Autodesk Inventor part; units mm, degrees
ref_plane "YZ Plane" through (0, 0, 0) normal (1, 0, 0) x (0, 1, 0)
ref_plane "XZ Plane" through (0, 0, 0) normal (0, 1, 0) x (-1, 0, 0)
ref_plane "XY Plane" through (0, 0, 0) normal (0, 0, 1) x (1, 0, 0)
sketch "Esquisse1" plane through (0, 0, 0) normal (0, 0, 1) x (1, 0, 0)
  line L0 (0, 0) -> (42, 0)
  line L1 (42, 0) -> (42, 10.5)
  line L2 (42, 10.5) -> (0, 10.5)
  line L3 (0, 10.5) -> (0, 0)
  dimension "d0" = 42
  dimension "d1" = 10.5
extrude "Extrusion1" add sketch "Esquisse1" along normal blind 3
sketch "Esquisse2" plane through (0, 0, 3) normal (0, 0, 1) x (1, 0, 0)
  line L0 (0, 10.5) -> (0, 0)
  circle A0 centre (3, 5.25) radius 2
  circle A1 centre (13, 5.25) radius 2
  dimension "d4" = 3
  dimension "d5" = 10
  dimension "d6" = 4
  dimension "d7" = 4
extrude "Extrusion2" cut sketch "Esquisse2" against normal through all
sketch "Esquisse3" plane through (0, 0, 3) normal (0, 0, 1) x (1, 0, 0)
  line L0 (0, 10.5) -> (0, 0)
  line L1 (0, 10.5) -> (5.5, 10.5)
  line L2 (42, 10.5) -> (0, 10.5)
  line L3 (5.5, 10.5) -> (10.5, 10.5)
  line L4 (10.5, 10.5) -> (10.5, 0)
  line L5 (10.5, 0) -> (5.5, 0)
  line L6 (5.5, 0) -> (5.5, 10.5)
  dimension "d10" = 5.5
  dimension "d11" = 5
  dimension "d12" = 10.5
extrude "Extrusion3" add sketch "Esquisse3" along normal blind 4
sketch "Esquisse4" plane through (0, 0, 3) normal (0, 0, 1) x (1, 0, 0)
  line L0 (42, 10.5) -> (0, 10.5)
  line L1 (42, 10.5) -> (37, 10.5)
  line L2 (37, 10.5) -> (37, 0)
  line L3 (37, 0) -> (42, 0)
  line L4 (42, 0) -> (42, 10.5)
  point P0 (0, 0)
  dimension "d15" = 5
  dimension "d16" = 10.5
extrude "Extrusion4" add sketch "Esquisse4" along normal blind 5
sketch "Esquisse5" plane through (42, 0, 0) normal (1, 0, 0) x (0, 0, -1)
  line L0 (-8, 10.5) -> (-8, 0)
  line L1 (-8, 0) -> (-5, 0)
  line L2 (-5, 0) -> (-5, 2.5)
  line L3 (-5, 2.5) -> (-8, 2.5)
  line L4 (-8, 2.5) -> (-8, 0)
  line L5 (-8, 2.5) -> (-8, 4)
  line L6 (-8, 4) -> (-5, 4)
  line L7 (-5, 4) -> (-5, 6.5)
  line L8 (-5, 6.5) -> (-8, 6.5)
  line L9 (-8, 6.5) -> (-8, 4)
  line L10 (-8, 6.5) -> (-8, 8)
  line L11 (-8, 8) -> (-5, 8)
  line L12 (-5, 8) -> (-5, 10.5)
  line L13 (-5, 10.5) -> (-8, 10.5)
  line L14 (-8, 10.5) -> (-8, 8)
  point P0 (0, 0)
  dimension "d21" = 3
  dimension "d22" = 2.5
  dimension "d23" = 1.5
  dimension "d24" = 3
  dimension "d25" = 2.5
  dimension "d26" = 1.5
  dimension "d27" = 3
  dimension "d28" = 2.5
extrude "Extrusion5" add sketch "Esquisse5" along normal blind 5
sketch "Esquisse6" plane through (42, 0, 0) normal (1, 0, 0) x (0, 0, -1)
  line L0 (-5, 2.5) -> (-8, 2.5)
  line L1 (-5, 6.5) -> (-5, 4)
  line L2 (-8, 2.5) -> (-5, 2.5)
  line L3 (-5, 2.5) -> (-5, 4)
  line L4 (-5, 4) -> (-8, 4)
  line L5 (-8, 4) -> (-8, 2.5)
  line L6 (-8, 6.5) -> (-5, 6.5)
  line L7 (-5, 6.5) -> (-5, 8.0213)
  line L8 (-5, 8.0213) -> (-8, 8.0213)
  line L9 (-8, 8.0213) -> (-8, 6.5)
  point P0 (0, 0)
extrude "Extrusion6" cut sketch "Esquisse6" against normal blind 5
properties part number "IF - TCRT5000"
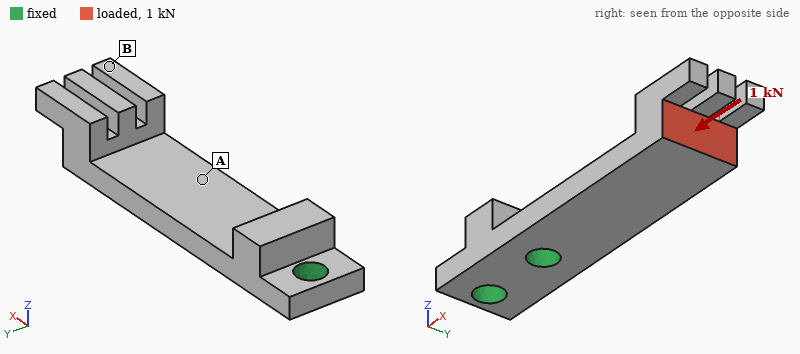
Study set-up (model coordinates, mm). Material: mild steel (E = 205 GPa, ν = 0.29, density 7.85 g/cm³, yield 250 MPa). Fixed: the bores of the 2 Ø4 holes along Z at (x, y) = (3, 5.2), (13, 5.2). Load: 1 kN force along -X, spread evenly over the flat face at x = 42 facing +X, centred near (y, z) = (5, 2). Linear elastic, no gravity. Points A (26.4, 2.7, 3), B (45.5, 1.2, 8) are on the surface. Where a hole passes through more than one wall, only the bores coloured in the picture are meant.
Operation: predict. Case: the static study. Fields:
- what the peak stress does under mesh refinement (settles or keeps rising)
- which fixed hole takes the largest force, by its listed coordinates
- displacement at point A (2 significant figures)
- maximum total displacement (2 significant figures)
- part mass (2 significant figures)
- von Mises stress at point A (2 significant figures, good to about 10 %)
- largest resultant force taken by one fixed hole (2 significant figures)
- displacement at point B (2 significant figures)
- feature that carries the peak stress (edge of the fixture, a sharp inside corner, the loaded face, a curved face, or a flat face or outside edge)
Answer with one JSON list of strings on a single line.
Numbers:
["keeps rising", "(13, 5.2)", "0.016 mm", "0.11 mm", "14 g", "95 MPa", "910 N", "0.10 mm", "edge of the fixture"]
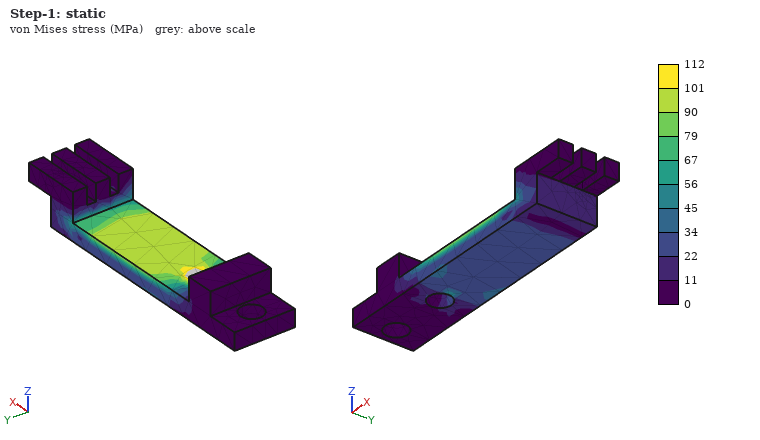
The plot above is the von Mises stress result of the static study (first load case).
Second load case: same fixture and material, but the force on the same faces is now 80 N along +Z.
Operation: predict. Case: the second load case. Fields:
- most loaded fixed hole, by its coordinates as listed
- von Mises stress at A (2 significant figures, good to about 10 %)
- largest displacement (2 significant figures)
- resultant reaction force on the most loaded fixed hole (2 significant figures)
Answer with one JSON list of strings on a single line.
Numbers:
["(13, 5.2)", "79 MPa", "0.15 mm", "98 N"]
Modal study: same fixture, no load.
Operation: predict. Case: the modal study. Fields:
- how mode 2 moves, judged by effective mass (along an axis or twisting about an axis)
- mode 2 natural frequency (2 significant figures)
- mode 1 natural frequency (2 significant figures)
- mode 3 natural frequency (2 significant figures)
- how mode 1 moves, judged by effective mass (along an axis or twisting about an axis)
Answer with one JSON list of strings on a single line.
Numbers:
["along Y", "5300 Hz", "2000 Hz", "9900 Hz", "along Z"]
